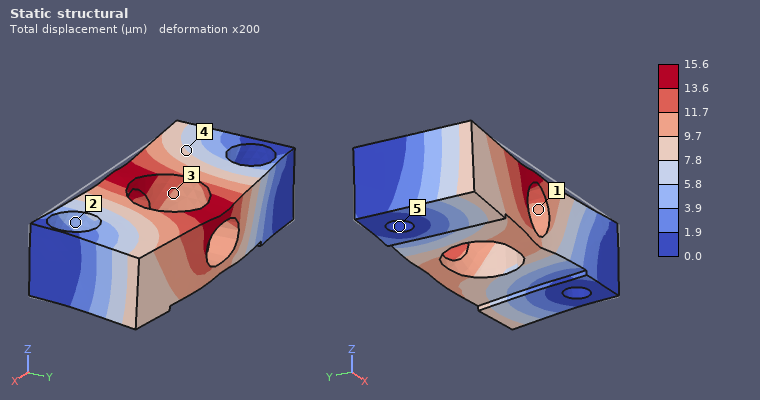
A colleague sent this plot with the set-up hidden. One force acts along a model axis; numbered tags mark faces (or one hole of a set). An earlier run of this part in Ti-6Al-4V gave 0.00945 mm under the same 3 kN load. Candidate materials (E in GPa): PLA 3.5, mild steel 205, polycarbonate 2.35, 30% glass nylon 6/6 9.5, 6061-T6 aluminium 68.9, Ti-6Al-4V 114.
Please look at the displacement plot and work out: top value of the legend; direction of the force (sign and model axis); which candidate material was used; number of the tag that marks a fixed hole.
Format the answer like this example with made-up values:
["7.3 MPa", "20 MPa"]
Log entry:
["15.6 µm", "+Y", "6061-T6 aluminium", "5"]
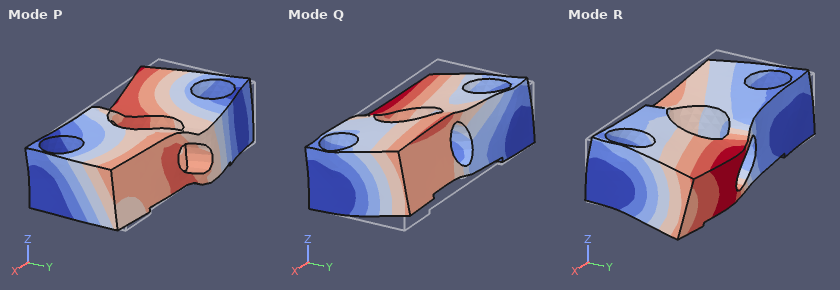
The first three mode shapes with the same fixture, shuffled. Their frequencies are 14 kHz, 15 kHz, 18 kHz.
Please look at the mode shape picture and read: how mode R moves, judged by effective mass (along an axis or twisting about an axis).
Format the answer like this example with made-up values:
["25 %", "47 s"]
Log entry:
["along Z"]
